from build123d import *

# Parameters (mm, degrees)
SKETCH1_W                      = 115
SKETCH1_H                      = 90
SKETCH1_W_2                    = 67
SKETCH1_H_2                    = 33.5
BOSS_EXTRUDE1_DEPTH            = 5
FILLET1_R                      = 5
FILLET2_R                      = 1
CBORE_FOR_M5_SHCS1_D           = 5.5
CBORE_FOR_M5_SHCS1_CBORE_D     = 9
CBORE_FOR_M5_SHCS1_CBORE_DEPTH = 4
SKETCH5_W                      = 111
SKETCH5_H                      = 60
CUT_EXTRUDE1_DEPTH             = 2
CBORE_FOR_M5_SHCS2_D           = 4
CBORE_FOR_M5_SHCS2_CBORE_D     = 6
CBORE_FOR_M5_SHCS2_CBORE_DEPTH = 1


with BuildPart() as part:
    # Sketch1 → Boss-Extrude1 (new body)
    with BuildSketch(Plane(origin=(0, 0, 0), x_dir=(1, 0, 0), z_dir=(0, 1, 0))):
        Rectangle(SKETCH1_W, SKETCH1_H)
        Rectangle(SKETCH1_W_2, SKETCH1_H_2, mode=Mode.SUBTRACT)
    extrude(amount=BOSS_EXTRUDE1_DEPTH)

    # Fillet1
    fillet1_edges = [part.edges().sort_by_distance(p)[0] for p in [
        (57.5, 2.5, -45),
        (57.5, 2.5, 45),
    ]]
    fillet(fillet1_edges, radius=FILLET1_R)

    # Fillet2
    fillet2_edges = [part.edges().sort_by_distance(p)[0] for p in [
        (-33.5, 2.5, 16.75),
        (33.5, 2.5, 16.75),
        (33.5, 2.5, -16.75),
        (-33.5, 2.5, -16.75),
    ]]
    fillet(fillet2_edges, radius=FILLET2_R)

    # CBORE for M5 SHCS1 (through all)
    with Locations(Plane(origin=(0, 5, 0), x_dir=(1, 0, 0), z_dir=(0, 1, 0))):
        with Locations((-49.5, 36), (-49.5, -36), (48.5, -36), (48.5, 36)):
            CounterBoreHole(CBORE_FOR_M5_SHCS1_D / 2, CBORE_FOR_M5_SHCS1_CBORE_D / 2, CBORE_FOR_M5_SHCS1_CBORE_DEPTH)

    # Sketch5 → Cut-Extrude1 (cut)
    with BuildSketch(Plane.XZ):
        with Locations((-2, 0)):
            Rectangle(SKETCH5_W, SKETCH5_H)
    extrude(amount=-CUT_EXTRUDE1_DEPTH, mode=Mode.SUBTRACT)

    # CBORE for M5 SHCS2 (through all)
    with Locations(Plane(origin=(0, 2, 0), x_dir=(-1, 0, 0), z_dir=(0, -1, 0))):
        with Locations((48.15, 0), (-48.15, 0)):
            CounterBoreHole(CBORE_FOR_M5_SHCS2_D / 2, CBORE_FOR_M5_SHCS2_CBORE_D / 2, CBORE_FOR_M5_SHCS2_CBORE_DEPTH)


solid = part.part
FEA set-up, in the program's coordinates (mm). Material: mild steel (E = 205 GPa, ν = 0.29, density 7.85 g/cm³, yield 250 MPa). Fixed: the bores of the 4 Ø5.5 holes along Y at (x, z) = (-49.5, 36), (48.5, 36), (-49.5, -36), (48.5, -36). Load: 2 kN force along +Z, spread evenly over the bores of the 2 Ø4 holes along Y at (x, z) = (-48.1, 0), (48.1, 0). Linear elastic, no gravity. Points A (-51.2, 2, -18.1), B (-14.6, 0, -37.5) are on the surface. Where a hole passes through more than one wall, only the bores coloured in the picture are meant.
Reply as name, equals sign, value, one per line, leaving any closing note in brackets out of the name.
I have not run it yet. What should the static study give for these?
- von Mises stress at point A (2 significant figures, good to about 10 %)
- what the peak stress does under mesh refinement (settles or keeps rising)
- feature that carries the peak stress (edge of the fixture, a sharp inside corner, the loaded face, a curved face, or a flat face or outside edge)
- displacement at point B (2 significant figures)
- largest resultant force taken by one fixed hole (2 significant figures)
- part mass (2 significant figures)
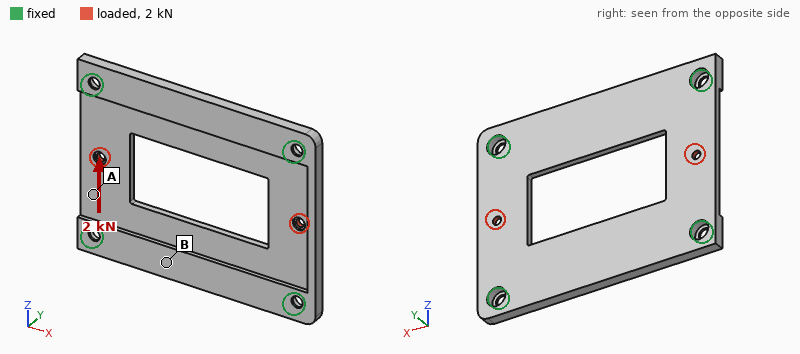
von Mises stress at point A = 16 MPa
what the peak stress does under mesh refinement = keeps rising
feature that carries the peak stress = edge of the fixture
displacement at point B = 1.5 µm
largest resultant force taken by one fixed hole = 520 N
part mass = 240 g
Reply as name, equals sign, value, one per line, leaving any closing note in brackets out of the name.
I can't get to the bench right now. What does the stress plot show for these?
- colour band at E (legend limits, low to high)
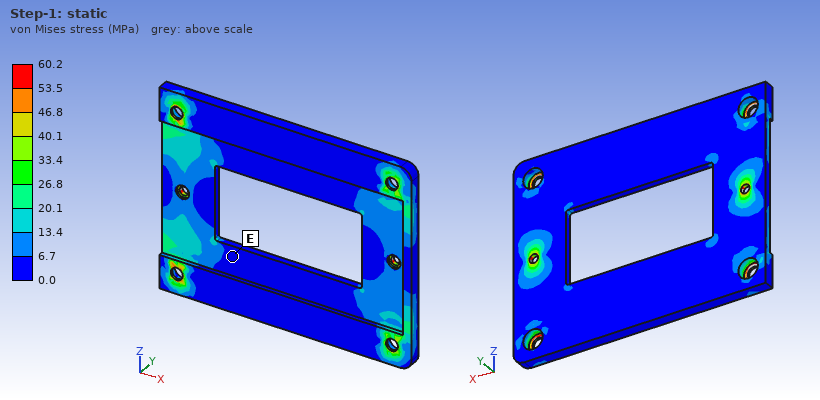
colour band at E = 0.0 to 6.7 MPa
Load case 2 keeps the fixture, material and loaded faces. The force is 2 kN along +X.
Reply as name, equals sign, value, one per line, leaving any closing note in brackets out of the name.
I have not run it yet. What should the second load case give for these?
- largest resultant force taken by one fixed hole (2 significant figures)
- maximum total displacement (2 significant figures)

largest resultant force taken by one fixed hole = 510 N
maximum total displacement = 9.1 µm
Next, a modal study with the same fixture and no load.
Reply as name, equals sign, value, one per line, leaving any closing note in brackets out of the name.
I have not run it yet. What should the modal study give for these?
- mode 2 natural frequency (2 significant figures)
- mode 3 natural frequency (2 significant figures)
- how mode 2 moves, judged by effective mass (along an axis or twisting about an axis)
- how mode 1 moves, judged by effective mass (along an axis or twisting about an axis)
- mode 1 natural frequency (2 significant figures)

mode 2 natural frequency = 2000 Hz
mode 3 natural frequency = 3200 Hz
how mode 2 moves, judged by effective mass = twisting about X
how mode 1 moves, judged by effective mass = along Y
mode 1 natural frequency = 1900 Hz
